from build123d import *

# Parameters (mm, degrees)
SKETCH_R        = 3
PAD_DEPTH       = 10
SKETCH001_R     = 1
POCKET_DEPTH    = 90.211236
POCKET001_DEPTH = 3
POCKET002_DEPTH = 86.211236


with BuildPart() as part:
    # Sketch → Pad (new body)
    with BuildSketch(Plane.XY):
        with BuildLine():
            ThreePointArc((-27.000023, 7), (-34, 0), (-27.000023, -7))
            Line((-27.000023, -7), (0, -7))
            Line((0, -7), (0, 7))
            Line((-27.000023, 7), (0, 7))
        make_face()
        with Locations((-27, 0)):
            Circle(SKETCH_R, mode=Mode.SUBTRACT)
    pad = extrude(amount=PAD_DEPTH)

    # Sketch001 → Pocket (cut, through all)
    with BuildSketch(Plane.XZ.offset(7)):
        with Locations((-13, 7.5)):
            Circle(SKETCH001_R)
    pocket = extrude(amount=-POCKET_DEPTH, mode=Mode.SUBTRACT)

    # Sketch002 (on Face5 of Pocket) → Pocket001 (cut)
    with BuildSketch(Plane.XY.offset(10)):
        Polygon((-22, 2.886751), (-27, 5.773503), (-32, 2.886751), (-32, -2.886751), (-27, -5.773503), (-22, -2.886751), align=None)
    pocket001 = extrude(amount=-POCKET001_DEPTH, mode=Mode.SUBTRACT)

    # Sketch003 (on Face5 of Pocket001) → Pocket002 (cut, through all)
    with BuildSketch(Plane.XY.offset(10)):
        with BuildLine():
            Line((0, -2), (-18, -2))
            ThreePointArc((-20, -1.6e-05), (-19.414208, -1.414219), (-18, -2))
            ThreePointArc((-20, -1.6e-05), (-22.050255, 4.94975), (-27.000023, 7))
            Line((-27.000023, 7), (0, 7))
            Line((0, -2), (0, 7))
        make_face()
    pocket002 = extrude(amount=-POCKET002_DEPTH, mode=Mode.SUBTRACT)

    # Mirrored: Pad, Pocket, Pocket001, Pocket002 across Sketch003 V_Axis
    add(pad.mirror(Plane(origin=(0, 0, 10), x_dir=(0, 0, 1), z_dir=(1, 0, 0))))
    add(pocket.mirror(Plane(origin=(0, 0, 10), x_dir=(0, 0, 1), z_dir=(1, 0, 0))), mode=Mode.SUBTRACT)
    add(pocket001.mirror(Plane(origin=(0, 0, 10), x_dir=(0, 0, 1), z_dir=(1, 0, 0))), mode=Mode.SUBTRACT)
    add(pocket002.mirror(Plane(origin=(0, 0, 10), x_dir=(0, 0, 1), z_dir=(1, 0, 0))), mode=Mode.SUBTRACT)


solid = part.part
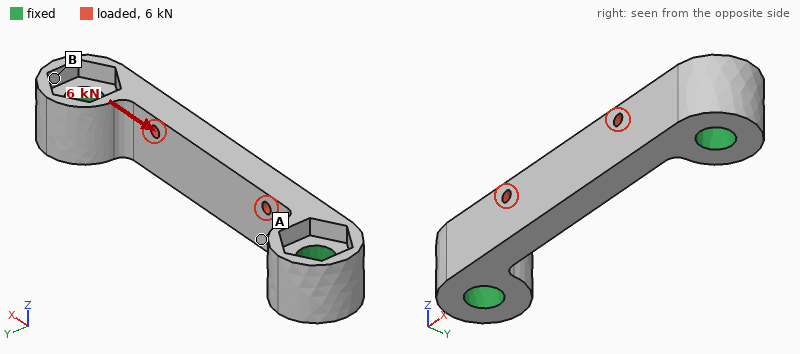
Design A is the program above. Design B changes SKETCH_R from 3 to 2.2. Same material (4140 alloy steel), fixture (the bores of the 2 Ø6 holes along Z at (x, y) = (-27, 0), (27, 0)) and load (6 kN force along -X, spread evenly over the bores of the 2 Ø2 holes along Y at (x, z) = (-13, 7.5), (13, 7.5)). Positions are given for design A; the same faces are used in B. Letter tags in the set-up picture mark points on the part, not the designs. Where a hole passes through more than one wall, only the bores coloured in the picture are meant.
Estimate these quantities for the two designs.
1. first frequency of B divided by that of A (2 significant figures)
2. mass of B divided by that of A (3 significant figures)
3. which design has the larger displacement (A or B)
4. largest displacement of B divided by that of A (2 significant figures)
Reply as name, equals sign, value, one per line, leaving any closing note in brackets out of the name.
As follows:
first frequency of B divided by that of A = 0.96
mass of B divided by that of A = 1.04
which design has the larger displacement = B
largest displacement of B divided by that of A = 1.2
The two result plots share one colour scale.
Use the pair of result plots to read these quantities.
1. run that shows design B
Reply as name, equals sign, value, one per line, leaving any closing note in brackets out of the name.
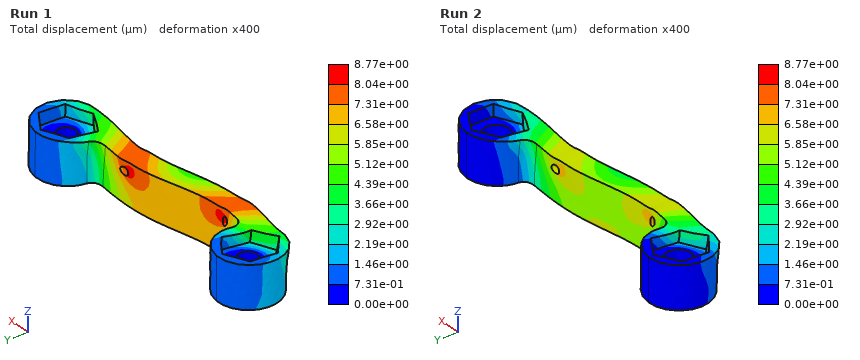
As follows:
run that shows design B = Run 1
